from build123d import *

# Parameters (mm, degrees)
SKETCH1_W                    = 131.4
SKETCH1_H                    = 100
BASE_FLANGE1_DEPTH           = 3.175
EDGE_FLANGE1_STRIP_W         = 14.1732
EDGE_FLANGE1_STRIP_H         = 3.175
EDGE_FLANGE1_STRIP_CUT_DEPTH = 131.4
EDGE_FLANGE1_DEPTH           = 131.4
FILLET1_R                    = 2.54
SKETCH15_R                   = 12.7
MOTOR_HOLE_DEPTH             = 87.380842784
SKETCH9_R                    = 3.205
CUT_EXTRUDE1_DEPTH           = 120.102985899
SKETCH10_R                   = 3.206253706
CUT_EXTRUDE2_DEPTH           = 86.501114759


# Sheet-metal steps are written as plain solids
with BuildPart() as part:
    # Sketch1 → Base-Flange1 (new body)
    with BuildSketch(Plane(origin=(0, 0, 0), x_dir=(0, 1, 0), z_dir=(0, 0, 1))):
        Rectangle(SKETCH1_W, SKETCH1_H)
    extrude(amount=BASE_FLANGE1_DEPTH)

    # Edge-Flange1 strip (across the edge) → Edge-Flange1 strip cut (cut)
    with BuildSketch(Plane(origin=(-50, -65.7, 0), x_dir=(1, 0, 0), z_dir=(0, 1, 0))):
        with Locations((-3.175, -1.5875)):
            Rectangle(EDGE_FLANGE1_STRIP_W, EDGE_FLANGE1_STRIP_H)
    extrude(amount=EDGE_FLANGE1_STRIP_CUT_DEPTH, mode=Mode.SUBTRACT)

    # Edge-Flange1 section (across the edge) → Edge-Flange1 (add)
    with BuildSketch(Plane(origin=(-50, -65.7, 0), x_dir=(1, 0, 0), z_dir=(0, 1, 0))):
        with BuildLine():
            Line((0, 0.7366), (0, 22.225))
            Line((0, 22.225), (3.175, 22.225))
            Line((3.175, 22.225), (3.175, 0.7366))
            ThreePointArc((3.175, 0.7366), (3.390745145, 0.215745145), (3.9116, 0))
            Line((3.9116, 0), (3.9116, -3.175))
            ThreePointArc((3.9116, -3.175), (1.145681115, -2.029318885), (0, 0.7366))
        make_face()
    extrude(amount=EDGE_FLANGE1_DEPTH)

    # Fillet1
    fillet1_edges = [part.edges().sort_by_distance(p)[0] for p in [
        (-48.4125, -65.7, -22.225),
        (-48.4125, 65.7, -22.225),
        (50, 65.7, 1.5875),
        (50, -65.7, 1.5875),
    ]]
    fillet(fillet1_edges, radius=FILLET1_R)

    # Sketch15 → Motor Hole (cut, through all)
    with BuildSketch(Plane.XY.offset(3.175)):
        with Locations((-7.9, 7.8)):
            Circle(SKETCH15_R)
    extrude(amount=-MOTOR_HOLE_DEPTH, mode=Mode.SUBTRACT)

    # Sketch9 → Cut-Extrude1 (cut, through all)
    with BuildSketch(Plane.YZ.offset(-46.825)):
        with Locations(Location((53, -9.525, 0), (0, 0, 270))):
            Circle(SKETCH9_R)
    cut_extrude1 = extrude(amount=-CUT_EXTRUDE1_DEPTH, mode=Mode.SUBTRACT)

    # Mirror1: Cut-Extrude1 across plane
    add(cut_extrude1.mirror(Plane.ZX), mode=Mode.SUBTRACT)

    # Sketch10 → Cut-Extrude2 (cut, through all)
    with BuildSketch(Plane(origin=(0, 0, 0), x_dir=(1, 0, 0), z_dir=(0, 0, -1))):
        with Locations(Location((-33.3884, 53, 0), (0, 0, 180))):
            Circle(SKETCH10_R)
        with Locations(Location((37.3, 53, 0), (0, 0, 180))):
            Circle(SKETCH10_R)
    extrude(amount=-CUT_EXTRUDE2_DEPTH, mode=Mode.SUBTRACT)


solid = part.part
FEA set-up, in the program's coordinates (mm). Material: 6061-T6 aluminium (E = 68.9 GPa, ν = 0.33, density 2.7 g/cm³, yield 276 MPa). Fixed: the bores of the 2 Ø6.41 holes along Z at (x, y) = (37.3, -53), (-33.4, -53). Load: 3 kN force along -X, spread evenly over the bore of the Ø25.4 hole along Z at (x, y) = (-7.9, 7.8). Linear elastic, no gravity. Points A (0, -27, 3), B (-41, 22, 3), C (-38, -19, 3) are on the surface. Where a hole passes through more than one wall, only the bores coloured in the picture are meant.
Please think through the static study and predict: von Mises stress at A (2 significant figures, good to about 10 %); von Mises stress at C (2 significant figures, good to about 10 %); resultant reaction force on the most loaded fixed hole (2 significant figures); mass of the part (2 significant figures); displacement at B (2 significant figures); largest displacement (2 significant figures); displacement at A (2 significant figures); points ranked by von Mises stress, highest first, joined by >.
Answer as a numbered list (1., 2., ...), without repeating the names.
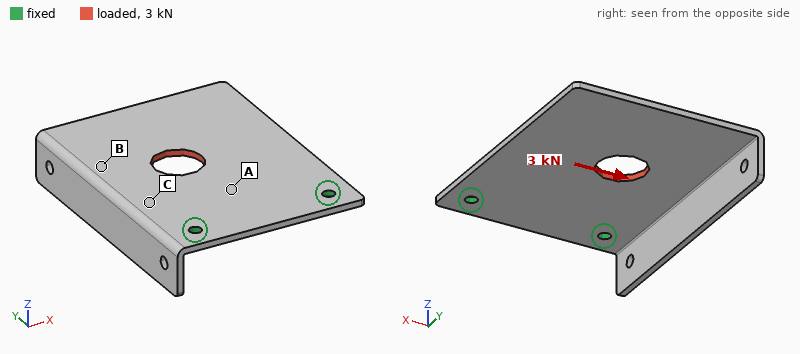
1. 26 MPa
2. 15 MPa
3. 2.9 kN
4. 130 g
5. 63 µm
6. 85 µm
7. 19 µm
8. A > C > B
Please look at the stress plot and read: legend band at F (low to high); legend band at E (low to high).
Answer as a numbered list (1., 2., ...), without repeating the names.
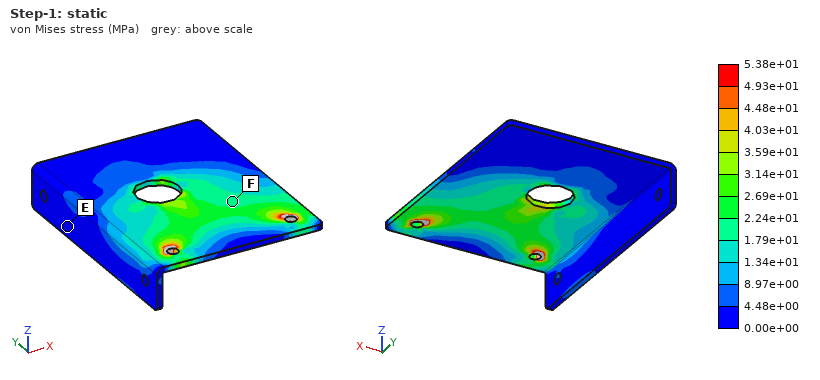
1. 1.79e+01 to 2.24e+01 MPa
2. 0.00e+00 to 4.48e+00 MPa
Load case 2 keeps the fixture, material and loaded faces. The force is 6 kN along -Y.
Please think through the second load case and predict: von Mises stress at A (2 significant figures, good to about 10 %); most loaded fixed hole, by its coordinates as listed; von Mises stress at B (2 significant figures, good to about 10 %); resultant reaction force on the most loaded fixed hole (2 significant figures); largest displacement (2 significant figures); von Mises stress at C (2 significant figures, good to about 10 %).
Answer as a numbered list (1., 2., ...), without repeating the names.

1. 15 MPa
2. (-33.4, -53)
3. 11 MPa
4. 3.8 kN
5. 79 µm
6. 26 MPa
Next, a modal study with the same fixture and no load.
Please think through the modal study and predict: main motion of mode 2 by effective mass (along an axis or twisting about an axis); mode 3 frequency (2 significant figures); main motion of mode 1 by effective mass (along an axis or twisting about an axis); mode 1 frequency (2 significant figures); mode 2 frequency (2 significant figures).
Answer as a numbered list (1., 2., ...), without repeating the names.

1. twisting about Y
2. 1300 Hz
3. along Z
4. 240 Hz
5. 470 Hz
